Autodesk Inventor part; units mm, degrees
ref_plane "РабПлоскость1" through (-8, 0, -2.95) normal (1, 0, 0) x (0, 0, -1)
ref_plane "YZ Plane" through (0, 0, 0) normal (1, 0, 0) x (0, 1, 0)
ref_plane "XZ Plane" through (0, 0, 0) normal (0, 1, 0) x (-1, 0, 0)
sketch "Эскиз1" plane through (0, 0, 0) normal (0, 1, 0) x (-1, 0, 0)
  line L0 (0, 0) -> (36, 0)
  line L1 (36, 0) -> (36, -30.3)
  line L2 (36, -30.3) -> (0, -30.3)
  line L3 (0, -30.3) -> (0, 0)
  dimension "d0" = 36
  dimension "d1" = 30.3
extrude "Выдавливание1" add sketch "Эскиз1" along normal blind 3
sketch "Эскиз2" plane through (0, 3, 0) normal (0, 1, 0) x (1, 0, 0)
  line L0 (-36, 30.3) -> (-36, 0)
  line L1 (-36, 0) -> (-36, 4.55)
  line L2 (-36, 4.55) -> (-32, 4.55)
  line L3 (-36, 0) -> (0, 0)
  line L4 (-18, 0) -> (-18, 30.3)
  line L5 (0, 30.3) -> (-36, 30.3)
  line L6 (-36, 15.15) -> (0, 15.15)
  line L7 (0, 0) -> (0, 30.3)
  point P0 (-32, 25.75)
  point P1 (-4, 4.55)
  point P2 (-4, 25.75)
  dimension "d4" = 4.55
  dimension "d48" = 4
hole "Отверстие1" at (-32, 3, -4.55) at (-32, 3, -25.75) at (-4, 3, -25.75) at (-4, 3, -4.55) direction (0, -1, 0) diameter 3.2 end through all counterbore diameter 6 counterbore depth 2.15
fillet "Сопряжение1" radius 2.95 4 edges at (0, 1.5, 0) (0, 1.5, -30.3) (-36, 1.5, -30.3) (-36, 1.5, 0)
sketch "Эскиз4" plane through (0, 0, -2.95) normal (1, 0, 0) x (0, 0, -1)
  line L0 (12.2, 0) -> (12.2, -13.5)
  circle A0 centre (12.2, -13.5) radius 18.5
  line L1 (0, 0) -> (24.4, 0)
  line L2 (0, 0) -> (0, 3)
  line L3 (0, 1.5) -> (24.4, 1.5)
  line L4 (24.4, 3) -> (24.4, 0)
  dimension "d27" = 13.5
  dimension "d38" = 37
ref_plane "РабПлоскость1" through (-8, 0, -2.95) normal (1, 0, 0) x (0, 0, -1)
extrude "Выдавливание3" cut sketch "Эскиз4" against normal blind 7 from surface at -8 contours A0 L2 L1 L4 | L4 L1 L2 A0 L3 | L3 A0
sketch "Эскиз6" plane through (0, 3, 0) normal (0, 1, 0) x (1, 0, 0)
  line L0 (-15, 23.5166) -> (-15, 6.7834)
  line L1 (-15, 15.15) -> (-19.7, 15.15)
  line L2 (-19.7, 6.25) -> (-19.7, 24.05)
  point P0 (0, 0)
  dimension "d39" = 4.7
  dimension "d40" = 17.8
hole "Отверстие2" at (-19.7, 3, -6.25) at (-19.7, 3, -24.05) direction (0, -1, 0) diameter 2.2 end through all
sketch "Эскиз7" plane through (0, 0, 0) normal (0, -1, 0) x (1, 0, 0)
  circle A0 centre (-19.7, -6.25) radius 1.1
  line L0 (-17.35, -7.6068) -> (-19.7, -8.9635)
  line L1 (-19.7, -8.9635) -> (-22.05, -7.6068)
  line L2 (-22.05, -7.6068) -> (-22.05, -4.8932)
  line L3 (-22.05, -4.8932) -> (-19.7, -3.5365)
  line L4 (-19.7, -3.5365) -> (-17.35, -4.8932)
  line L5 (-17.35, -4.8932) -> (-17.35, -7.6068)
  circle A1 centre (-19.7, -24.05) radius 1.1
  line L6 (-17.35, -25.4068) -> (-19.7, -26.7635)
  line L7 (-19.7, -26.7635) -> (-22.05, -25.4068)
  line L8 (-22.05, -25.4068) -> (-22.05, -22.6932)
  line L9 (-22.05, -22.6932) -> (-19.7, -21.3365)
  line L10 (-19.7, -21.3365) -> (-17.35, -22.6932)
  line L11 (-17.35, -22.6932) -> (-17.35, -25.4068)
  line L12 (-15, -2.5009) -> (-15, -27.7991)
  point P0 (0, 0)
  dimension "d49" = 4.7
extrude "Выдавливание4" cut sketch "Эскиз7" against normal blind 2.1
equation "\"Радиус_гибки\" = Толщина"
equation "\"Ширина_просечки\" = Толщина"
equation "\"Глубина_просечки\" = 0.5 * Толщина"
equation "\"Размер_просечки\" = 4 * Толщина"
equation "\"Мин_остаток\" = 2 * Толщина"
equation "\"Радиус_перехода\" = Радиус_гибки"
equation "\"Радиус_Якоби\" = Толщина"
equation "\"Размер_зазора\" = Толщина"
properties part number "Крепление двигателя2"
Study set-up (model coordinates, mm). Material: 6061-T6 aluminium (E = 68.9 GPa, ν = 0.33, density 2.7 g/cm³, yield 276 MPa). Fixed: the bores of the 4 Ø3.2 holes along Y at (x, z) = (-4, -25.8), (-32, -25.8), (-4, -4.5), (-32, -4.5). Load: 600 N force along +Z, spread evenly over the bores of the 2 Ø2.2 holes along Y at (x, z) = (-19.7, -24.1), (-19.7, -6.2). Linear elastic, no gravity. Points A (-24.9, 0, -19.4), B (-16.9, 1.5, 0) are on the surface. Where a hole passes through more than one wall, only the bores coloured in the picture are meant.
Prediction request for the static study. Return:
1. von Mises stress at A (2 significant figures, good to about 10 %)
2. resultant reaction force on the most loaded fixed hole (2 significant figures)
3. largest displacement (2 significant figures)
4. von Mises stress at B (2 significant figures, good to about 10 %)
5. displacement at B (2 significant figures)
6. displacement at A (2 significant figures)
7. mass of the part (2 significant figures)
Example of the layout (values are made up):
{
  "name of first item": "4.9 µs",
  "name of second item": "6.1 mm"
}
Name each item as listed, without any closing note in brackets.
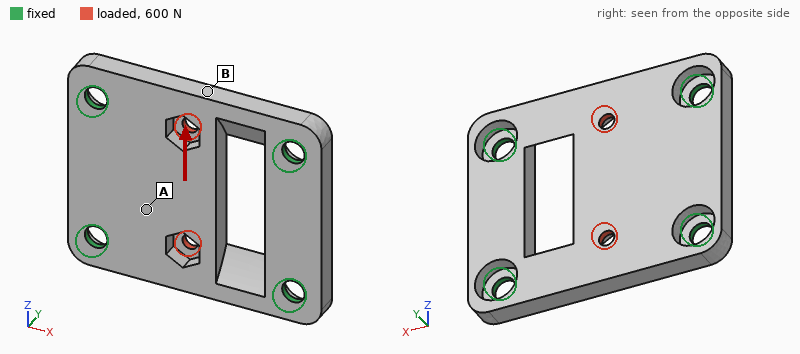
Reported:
{
  "von Mises stress at A": "11 MPa",
  "resultant reaction force on the most loaded fixed hole": "310 N",
  "largest displacement": "8.0 µm",
  "von Mises stress at B": "22 MPa",
  "displacement at B": "6.6 µm",
  "displacement at A": "3.7 µm",
  "mass of the part": "6.6 g"
}
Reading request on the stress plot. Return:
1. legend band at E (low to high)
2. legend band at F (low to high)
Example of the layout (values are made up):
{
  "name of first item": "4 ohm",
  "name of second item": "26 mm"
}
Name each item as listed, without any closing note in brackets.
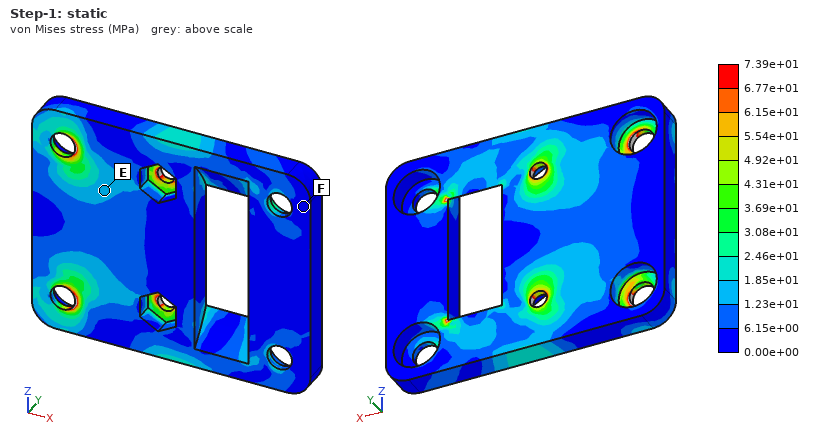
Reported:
{
  "legend band at E": "1.23e+01 to 1.85e+01 MPa",
  "legend band at F": "0.00e+00 to 6.15e+00 MPa"
}
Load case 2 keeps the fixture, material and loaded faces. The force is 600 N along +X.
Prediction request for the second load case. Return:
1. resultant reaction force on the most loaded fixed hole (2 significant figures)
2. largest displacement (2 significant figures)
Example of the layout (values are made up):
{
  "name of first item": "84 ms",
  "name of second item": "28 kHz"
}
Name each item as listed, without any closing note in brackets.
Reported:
{
  "resultant reaction force on the most loaded fixed hole": "210 N",
  "largest displacement": "9.1 µm"
}
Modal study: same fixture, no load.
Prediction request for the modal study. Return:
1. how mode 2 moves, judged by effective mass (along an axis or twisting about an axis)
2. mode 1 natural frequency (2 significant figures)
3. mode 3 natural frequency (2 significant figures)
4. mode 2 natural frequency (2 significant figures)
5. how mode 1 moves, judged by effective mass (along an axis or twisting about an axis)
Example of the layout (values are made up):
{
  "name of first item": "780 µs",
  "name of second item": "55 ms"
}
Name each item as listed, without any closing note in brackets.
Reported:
{
  "how mode 2 moves, judged by effective mass": "twisting about X",
  "mode 1 natural frequency": "10 kHz",
  "mode 3 natural frequency": "21 kHz",
  "mode 2 natural frequency": "16 kHz",
  "how mode 1 moves, judged by effective mass": "along Y"
}
